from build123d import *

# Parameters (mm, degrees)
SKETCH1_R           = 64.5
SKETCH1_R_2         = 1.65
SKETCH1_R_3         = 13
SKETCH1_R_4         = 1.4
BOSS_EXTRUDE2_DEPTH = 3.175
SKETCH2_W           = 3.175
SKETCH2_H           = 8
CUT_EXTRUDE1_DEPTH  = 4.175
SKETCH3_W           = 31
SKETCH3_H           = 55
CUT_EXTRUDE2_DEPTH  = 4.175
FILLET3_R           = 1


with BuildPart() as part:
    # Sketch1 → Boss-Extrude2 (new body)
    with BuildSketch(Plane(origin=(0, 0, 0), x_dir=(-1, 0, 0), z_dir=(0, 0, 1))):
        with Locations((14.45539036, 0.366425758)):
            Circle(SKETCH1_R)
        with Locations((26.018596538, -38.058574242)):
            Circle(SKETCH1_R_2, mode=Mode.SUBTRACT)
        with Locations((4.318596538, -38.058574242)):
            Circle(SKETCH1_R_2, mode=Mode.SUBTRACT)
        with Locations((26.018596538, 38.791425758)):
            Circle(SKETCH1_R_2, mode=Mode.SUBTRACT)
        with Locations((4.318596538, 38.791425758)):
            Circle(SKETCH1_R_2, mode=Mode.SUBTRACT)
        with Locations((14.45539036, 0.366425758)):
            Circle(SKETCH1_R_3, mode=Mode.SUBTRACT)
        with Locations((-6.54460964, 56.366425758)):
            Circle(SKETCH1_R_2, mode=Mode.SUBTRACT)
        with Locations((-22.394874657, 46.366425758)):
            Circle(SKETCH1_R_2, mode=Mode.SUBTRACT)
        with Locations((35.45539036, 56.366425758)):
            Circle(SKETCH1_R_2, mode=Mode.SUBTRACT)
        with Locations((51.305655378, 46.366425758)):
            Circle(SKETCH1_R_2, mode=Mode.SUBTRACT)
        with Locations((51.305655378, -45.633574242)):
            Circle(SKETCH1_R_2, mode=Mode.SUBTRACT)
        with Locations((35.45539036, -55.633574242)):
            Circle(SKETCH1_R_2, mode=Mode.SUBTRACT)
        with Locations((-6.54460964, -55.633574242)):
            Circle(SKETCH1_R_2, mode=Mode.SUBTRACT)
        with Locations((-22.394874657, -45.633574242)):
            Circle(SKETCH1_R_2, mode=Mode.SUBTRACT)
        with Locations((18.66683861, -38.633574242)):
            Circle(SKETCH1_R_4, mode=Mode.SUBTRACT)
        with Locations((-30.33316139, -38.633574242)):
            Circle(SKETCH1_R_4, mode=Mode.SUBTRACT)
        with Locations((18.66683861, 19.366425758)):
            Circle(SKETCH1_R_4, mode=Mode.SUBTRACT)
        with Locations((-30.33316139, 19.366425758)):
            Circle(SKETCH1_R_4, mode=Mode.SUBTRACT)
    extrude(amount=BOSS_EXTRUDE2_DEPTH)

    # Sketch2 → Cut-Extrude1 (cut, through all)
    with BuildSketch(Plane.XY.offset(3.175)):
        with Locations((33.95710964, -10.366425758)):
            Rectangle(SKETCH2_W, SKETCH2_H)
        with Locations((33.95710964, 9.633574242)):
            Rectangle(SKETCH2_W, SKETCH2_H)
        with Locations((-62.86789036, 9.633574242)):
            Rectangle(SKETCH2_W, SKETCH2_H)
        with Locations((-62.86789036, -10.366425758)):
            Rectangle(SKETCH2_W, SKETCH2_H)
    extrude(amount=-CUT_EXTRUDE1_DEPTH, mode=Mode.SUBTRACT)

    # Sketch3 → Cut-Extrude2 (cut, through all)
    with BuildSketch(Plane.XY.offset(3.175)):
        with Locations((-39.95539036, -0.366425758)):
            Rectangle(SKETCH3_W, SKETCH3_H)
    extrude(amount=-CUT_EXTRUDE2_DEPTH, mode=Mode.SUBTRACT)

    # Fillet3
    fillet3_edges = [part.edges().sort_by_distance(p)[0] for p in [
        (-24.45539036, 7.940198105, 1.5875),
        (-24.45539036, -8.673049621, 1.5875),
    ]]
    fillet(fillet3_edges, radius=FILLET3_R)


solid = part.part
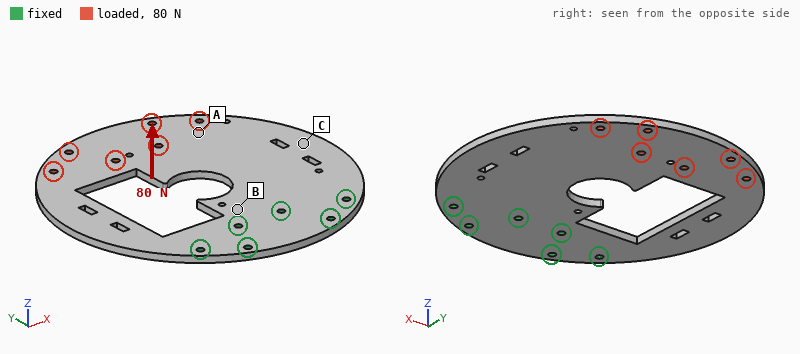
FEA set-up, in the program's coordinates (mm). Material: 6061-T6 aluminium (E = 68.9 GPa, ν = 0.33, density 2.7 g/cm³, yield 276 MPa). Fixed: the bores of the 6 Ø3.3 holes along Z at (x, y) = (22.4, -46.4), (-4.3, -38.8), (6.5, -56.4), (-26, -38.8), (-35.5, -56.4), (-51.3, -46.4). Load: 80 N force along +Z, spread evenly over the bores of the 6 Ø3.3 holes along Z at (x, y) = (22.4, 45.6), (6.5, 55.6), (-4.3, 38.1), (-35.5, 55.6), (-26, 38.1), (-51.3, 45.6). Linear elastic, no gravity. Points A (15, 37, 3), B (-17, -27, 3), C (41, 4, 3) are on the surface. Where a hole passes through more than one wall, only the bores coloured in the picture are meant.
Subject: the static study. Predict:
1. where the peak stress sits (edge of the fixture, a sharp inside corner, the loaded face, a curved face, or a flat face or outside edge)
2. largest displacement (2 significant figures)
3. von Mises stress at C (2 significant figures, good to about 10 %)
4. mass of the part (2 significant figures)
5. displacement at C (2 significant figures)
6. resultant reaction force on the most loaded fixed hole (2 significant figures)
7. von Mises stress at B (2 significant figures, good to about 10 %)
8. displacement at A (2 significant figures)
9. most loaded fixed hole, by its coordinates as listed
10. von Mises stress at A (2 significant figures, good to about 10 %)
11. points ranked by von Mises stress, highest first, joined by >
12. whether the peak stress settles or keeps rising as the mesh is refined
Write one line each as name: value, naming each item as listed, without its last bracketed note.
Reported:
where the peak stress sits: edge of the fixture
largest displacement: 1.9 mm
von Mises stress at C: 24 MPa
mass of the part: 91 g
displacement at C: 0.44 mm
resultant reaction force on the most loaded fixed hole: 160 N
von Mises stress at B: 37 MPa
displacement at A: 1.1 mm
most loaded fixed hole, by its coordinates as listed: (-4.3, -38.8)
von Mises stress at A: 11 MPa
points ranked by von Mises stress, highest first, joined by >: B > C > A
whether the peak stress settles or keeps rising as the mesh is refined: keeps rising
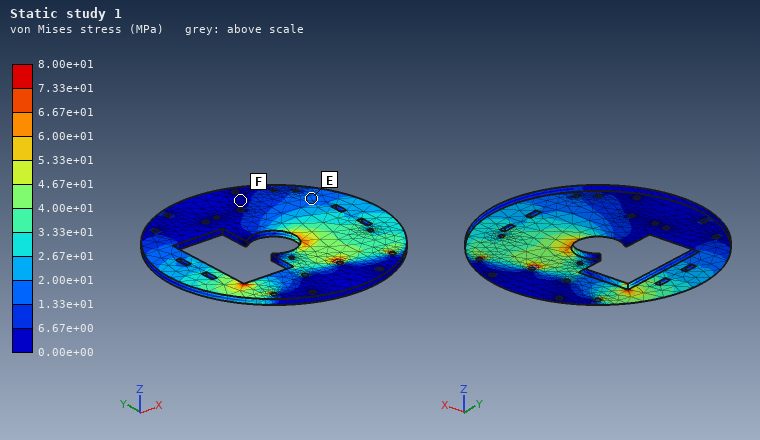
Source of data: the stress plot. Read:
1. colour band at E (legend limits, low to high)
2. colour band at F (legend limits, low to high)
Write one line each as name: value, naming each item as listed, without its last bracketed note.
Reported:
colour band at E: 1.33e+01 to 2.00e+01 MPa
colour band at F: 0.00e+00 to 6.67e+00 MPa
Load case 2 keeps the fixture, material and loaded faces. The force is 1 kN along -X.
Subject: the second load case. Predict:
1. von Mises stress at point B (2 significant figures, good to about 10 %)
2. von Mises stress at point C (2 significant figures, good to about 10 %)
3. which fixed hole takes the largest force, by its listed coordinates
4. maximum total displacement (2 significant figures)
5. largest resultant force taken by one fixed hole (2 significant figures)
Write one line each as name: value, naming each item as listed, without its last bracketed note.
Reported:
von Mises stress at point B: 22 MPa
von Mises stress at point C: 8.0 MPa
which fixed hole takes the largest force, by its listed coordinates: (22.4, -46.4)
maximum total displacement: 76 µm
largest resultant force taken by one fixed hole: 1.4 kN
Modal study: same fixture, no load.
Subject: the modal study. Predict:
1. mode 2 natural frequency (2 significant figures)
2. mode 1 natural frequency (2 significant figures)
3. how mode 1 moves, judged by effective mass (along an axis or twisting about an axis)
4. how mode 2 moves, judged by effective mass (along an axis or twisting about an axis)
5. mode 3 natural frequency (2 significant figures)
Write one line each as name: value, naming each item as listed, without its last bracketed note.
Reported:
mode 2 natural frequency: 500 Hz
mode 1 natural frequency: 220 Hz
how mode 1 moves, judged by effective mass: along Z
how mode 2 moves, judged by effective mass: twisting about Y
mode 3 natural frequency: 1100 Hz
